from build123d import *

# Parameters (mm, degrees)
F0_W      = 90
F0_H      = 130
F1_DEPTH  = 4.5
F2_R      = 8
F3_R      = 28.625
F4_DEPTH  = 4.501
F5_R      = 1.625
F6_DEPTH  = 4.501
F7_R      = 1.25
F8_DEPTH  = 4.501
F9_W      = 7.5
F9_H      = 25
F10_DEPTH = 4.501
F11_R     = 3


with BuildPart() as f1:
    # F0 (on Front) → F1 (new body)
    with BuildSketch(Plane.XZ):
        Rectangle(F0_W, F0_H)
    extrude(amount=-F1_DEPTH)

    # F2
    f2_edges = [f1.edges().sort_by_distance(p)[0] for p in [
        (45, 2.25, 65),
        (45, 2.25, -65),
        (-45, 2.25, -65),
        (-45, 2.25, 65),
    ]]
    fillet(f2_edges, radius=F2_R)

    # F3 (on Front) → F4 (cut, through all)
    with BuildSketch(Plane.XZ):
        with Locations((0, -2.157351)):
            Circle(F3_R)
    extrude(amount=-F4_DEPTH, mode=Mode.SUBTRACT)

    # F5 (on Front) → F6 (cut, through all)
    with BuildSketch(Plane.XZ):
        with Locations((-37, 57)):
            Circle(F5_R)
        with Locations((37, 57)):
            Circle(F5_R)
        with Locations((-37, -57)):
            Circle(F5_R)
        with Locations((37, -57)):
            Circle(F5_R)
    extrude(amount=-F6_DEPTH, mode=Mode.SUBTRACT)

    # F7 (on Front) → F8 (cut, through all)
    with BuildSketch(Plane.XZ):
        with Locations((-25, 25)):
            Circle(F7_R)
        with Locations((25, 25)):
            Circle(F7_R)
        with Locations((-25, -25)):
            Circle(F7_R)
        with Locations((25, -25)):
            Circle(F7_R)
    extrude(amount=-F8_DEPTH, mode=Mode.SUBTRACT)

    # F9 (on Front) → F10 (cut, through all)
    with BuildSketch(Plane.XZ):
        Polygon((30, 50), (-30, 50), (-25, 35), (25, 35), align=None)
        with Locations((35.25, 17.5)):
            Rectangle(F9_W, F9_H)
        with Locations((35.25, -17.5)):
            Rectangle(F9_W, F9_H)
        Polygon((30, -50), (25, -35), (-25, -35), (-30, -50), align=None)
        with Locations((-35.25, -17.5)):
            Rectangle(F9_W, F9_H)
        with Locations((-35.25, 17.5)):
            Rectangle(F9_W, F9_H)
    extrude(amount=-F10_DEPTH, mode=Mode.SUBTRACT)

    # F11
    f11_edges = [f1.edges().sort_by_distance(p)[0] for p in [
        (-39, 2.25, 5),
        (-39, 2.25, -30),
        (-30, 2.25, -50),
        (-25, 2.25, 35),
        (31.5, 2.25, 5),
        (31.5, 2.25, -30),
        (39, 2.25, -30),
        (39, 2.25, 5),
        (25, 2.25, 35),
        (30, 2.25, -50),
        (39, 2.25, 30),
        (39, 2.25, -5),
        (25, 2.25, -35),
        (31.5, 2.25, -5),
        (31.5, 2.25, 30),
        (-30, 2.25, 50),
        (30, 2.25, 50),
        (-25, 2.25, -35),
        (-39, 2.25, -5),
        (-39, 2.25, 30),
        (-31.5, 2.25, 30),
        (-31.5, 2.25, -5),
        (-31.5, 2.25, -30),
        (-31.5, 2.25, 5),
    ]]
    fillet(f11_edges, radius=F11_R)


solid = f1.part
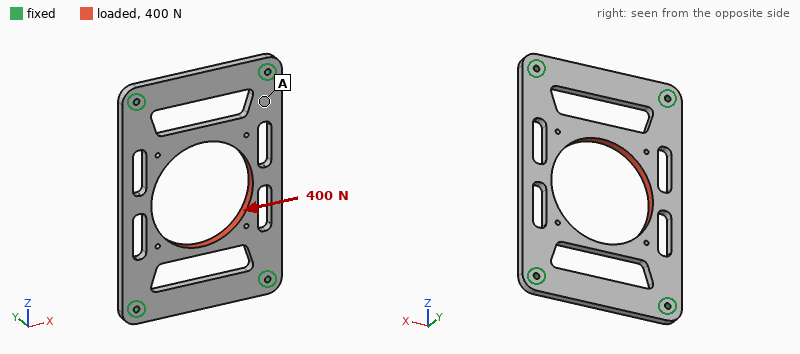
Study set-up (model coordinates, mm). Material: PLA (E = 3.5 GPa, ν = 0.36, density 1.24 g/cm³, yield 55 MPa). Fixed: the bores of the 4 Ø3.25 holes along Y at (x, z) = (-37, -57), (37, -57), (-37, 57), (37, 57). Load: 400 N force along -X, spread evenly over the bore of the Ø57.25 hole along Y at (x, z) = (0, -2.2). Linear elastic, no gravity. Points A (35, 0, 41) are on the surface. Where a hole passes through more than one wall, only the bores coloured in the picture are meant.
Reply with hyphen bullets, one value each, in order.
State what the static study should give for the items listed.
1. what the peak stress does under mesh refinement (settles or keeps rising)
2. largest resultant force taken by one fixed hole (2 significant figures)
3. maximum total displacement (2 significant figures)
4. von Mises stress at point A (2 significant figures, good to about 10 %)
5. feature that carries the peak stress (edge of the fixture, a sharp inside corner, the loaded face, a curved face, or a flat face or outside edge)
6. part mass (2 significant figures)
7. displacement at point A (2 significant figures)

- keeps rising
- 120 N
- 0.23 mm
- 3.4 MPa
- edge of the fixture
- 37 g
- 0.063 mm
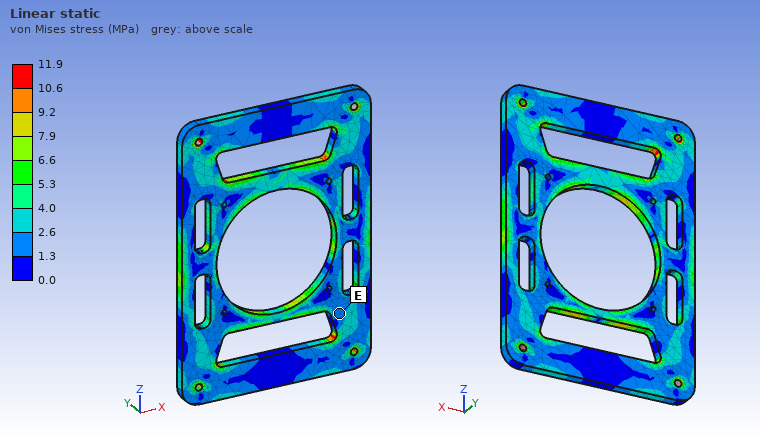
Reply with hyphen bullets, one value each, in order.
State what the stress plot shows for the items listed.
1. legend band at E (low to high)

- 1.3 to 2.6 MPa
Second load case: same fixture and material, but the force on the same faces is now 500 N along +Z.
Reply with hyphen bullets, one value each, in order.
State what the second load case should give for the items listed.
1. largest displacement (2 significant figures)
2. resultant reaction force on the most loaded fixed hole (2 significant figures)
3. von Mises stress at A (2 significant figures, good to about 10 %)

- 0.17 mm
- 130 N
- 1.4 MPa
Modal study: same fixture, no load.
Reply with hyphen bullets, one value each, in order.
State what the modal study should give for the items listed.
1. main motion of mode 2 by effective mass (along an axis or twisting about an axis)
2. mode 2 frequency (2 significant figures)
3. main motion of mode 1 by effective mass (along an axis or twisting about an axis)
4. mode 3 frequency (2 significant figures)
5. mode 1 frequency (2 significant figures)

- twisting about Z
- 680 Hz
- along Y
- 1000 Hz
- 540 Hz
